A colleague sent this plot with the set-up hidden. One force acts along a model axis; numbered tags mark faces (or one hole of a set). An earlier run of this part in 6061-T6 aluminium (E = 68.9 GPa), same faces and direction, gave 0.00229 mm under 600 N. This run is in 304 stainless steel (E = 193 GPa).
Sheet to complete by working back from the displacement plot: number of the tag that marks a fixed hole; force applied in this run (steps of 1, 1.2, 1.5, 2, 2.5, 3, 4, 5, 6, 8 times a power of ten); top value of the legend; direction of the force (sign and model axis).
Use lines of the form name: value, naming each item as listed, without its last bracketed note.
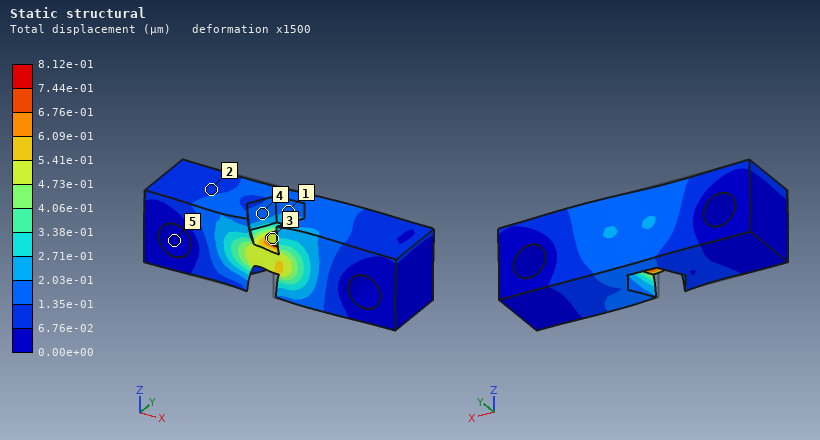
number of the tag that marks a fixed hole: 5
force applied in this run: 600 N
top value of the legend: 8.12e-01 µm
direction of the force: +X
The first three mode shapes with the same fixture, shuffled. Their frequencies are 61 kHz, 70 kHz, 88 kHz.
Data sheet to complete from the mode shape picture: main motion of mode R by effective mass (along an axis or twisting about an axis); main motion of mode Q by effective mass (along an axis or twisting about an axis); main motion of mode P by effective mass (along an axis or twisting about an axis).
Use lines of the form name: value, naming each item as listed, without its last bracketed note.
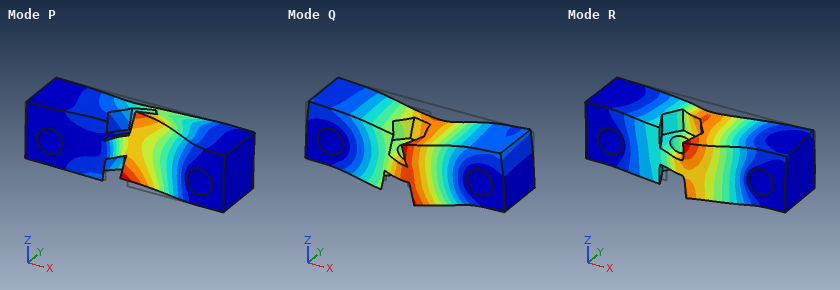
main motion of mode R by effective mass: along Y
main motion of mode Q by effective mass: along Z
main motion of mode P by effective mass: twisting about X
